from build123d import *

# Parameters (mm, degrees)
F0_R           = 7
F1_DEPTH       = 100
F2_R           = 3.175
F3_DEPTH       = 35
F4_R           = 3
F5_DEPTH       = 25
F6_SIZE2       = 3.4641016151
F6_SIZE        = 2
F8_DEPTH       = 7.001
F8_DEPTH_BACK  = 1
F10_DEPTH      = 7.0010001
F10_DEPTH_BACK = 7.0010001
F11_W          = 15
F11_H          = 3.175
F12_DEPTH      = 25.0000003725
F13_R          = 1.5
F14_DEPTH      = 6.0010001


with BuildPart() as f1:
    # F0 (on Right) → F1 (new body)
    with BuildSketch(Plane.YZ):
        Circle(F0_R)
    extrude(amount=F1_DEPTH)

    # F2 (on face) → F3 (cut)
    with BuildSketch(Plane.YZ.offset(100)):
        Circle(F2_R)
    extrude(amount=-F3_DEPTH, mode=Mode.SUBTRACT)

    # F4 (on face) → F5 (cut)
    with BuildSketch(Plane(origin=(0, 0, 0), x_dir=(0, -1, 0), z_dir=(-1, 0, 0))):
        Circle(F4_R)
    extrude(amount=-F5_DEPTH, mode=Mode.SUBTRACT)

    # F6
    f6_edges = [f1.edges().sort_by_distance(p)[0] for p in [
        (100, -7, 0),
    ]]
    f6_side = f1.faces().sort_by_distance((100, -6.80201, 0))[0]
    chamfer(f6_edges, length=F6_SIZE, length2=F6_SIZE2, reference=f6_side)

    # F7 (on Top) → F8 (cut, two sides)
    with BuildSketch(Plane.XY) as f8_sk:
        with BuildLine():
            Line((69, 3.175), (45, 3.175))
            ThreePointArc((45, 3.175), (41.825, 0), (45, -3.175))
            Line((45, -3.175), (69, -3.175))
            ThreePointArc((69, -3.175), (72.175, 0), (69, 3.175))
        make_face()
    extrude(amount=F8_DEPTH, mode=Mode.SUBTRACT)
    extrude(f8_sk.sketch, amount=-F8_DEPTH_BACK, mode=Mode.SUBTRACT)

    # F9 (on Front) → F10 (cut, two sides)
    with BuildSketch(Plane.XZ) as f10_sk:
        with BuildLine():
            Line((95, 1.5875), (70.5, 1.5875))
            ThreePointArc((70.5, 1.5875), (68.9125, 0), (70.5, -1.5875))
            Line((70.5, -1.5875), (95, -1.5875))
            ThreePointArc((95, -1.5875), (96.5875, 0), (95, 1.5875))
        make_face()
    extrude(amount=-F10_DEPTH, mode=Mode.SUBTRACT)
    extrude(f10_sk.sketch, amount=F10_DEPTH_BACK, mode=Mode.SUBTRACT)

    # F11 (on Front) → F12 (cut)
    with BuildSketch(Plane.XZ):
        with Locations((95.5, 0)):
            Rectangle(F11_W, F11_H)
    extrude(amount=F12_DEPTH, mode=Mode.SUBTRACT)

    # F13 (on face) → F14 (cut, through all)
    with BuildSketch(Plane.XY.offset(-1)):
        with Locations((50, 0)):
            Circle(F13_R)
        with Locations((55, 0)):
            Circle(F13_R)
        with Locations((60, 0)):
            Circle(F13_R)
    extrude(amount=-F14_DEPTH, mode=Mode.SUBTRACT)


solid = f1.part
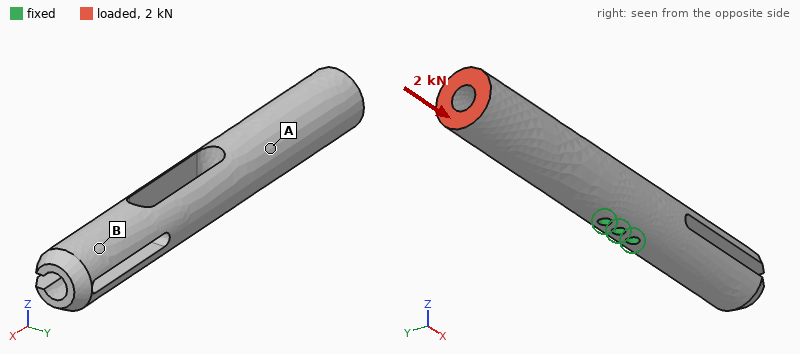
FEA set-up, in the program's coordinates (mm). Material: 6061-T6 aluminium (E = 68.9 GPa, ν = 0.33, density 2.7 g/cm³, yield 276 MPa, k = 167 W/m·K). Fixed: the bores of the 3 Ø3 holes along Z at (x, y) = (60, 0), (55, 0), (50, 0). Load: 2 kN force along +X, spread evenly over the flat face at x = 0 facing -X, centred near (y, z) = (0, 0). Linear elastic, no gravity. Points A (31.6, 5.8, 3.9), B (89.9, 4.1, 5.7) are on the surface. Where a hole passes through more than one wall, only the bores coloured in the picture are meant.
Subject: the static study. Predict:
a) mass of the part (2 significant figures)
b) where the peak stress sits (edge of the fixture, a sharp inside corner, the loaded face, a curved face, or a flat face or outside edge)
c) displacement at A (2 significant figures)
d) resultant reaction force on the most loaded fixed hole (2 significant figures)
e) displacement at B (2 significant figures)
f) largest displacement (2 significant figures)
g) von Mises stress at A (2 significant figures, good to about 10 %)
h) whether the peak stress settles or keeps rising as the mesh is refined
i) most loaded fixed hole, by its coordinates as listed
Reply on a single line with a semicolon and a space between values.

31 g; edge of the fixture; 19 µm; 1.2 kN; 10.0 µm; 49 µm; 14 MPa; keeps rising; (50, 0)
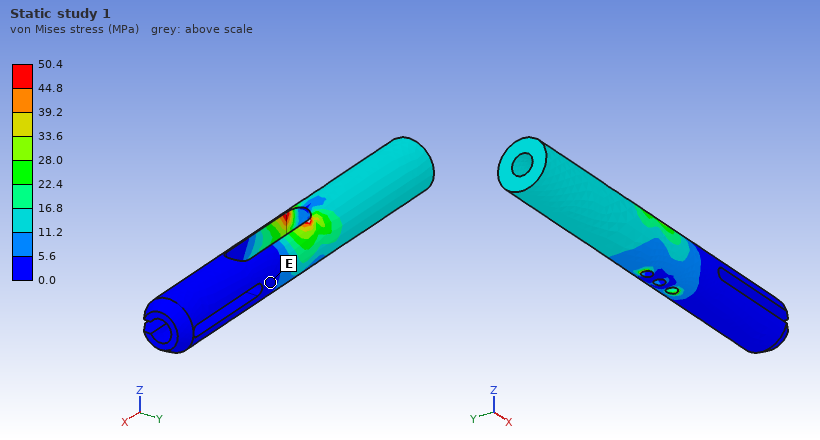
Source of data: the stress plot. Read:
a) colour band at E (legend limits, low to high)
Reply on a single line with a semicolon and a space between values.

0.0 to 5.6 MPa
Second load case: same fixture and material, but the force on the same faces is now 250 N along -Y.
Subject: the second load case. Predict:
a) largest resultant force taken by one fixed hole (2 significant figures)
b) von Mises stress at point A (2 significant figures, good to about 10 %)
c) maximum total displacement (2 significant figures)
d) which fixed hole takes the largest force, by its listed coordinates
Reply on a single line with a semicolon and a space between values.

1.1 kN; 25 MPa; 0.14 mm; (50, 0)
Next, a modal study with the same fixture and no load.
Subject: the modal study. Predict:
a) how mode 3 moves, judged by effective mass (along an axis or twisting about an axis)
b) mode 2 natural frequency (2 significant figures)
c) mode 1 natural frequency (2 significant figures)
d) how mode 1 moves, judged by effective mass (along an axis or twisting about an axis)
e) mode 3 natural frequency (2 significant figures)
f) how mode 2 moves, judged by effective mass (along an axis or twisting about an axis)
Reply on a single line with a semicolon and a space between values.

along Z; 3100 Hz; 2900 Hz; along Z; 3500 Hz; along Y
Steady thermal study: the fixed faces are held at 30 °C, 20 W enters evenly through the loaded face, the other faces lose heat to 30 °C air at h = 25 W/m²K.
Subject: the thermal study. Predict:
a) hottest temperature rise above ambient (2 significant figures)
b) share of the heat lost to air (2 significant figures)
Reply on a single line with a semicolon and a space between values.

46 K; 9.0 %
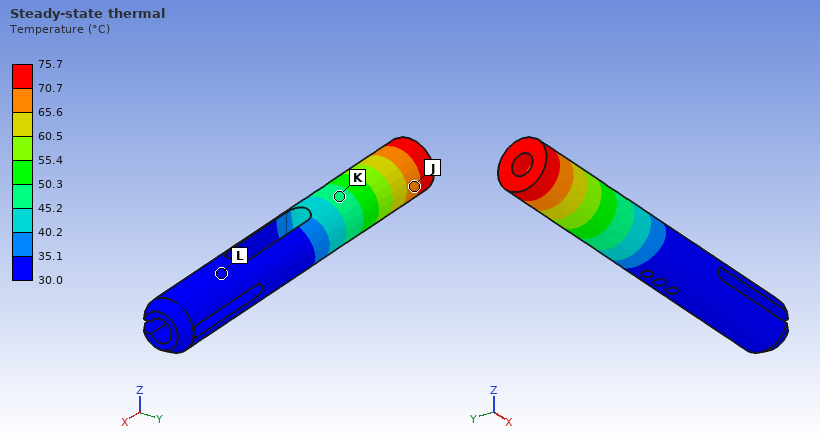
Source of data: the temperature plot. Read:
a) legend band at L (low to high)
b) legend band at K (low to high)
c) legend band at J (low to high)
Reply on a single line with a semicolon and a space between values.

30.0 to 35.1 °C; 45.2 to 50.3 °C; 65.6 to 70.7 °C
